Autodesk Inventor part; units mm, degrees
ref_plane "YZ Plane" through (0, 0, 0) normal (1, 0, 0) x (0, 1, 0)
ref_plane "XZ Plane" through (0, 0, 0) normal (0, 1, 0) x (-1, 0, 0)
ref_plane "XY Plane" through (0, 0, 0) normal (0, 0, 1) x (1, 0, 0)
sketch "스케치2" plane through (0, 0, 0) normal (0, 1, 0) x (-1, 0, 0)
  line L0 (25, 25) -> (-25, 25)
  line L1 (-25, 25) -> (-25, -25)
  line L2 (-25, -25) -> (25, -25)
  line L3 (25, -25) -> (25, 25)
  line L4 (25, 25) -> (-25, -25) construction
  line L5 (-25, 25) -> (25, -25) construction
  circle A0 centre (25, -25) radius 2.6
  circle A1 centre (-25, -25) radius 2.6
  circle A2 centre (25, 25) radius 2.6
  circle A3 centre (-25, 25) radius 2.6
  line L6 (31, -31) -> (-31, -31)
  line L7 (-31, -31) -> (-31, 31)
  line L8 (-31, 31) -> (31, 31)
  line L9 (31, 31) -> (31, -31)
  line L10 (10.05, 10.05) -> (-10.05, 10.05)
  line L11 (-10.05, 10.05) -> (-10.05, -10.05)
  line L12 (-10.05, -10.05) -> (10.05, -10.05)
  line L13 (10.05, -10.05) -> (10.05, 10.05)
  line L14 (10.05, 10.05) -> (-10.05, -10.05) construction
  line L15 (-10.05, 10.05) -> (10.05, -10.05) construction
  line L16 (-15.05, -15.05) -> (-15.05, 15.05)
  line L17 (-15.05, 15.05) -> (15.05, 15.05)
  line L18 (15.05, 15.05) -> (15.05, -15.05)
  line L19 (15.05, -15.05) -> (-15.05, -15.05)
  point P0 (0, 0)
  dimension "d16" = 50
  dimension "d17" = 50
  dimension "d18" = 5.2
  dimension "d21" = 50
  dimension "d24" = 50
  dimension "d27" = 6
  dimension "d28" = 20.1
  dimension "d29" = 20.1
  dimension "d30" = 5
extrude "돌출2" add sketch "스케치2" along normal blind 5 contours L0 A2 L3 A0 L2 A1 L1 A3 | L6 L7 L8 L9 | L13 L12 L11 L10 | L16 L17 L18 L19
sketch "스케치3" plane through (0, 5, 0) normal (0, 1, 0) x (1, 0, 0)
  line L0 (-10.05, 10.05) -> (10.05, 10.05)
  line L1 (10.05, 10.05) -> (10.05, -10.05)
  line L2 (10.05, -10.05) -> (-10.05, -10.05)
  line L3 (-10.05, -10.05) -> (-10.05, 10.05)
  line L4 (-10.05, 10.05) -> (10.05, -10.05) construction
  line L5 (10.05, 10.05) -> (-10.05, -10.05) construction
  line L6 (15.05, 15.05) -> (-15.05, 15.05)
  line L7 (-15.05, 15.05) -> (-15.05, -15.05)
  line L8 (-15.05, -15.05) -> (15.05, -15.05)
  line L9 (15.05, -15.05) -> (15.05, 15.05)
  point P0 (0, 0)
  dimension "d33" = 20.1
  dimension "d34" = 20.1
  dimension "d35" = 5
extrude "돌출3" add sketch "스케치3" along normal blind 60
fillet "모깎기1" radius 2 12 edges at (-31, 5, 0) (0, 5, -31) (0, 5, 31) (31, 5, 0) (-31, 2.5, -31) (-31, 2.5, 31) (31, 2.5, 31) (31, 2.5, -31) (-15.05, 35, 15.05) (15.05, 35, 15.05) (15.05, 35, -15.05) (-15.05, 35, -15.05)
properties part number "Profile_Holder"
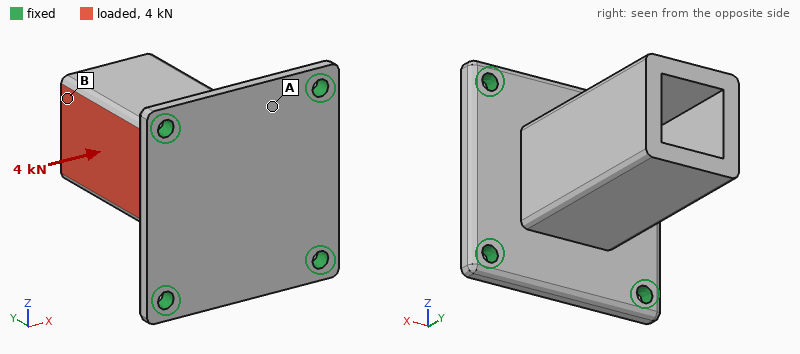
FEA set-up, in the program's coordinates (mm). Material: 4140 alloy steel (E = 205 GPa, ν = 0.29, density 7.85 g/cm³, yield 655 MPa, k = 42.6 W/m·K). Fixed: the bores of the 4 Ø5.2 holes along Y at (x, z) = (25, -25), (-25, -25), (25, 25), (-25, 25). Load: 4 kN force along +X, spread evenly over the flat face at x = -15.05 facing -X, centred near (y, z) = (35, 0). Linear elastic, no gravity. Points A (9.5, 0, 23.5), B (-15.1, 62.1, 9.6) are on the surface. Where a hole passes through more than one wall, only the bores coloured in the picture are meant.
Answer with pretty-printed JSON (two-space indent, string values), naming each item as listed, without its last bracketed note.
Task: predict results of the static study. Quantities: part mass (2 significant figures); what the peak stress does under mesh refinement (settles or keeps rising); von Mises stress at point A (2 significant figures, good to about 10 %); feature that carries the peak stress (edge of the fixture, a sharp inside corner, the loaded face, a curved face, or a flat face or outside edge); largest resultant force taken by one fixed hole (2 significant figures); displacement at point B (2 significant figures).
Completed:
{
  "part mass": "380 g",
  "what the peak stress does under mesh refinement": "keeps rising",
  "von Mises stress at point A": "45 MPa",
  "feature that carries the peak stress": "edge of the fixture",
  "largest resultant force taken by one fixed hole": "1.9 kN",
  "displacement at point B": "88 µm"
}
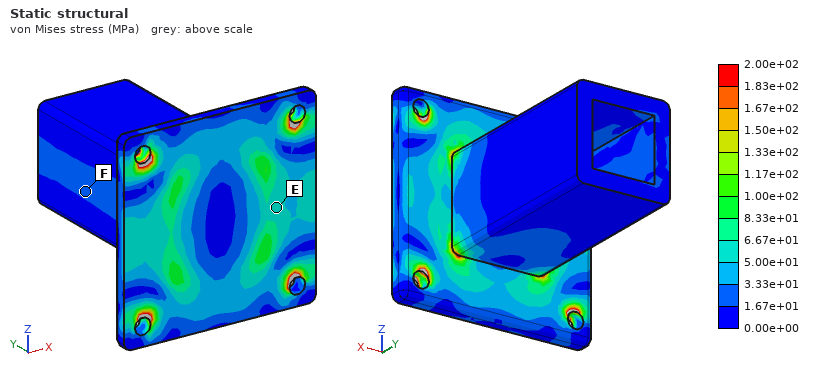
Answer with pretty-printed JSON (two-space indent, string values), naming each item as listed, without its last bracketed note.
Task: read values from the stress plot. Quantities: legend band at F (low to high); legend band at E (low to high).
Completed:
{
  "legend band at F": "1.67e+01 to 3.33e+01 MPa",
  "legend band at E": "5.00e+01 to 6.67e+01 MPa"
}
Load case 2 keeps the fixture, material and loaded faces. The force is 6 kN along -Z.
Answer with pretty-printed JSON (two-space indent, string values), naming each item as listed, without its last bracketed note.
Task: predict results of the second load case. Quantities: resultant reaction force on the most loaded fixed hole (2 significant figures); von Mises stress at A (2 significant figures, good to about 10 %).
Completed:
{
  "resultant reaction force on the most loaded fixed hole": "3.2 kN",
  "von Mises stress at A": "56 MPa"
}
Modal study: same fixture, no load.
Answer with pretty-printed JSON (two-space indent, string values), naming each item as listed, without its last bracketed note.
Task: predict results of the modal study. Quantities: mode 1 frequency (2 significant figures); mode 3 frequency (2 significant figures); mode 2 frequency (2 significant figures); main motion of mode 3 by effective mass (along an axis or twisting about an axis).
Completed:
{
  "mode 1 frequency": "2600 Hz",
  "mode 3 frequency": "4600 Hz",
  "mode 2 frequency": "2600 Hz",
  "main motion of mode 3 by effective mass": "along Y"
}
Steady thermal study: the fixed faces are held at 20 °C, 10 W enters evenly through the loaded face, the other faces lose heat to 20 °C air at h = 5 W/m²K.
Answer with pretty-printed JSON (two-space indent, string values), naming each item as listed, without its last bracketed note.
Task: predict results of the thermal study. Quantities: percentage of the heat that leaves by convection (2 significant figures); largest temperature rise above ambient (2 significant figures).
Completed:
{
  "percentage of the heat that leaves by convection": "12 %",
  "largest temperature rise above ambient": "26 K"
}
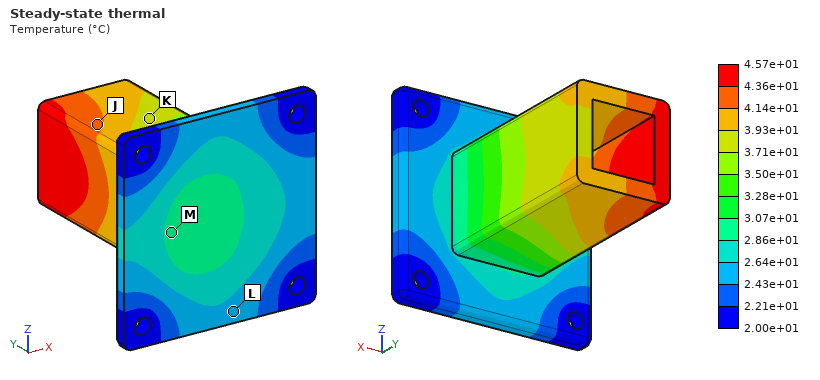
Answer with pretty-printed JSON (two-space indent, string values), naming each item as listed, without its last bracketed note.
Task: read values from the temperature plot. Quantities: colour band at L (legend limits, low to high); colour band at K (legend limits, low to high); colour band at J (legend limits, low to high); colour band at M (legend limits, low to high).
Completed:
{
  "colour band at L": "2.43e+01 to 2.64e+01 °C",
  "colour band at K": "3.71e+01 to 3.93e+01 °C",
  "colour band at J": "4.14e+01 to 4.36e+01 °C",
  "colour band at M": "2.86e+01 to 3.07e+01 °C"
}
